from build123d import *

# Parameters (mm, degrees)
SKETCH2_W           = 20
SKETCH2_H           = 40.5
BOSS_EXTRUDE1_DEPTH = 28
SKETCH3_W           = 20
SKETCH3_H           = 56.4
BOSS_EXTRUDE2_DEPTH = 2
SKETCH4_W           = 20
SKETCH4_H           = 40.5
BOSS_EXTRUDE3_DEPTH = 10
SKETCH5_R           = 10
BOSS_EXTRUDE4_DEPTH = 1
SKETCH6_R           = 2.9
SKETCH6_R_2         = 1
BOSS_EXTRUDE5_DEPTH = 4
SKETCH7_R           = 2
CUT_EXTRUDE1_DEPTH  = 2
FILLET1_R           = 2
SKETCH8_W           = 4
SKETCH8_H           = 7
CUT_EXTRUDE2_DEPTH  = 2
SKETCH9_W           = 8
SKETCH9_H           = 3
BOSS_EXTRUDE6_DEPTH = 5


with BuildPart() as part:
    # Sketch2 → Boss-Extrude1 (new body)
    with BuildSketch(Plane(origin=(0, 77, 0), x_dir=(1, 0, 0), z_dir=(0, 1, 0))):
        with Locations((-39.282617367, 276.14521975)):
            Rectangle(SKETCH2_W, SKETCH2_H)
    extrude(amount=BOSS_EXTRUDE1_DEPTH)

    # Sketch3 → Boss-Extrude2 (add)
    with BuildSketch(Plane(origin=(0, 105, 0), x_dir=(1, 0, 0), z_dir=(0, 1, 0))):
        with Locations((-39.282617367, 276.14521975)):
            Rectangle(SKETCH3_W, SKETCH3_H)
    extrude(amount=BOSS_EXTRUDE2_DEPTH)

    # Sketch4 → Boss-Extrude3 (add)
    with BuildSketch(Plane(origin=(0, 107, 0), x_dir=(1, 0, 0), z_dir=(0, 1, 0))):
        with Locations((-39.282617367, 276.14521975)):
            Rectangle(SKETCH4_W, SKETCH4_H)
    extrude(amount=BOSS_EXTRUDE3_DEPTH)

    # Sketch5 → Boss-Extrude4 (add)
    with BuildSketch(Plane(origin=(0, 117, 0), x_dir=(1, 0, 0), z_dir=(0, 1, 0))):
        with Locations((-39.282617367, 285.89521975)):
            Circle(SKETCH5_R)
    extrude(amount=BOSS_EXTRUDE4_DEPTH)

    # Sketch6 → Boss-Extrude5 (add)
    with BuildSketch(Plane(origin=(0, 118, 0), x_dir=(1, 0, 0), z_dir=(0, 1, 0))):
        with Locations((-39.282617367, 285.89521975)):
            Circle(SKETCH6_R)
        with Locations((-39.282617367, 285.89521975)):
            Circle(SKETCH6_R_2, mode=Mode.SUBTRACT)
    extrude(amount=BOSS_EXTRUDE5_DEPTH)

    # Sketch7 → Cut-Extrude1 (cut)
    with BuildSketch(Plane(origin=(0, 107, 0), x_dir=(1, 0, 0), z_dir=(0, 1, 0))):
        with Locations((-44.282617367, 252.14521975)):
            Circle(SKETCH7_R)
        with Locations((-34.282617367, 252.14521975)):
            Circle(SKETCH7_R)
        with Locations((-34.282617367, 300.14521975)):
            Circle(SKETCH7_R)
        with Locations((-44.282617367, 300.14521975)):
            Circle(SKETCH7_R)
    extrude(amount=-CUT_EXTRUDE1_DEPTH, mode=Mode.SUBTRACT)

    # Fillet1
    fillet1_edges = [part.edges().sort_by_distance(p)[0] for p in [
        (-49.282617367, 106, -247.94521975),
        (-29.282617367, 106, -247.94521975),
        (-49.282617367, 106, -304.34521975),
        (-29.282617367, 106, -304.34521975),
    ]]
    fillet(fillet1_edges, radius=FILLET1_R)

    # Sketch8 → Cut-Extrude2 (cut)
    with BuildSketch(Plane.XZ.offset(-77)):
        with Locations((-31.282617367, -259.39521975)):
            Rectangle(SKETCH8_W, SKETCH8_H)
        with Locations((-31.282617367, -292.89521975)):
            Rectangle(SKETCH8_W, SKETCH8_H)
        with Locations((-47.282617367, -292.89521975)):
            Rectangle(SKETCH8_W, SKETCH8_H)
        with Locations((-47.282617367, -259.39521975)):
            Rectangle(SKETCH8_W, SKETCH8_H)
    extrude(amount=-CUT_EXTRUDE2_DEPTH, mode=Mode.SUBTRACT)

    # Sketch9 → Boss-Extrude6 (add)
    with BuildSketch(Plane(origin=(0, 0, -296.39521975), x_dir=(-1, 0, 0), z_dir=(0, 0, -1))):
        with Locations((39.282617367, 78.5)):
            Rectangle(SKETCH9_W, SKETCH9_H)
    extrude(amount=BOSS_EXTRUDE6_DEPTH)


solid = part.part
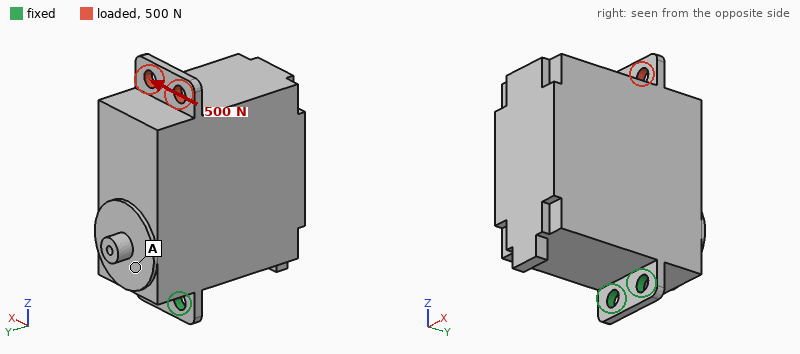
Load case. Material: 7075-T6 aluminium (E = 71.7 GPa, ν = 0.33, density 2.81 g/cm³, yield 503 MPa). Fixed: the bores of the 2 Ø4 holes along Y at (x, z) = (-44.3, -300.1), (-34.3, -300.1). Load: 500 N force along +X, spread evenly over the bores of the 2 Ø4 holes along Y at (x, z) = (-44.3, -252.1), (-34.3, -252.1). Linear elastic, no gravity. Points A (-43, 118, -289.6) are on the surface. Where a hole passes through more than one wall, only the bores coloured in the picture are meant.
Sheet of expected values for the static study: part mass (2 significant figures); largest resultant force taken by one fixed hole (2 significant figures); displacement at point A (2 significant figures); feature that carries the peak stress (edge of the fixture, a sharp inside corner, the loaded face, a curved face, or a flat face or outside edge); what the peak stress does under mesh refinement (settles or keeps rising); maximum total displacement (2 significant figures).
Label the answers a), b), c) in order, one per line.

a) 93 g
b) 1.9 kN
c) 15 µm
d) edge of the fixture
e) keeps rising
f) 96 µm
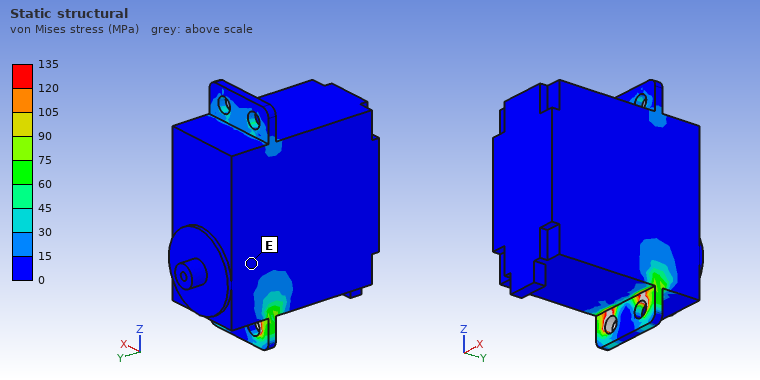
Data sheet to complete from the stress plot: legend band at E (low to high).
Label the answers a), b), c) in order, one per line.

a) 0 to 15 MPa
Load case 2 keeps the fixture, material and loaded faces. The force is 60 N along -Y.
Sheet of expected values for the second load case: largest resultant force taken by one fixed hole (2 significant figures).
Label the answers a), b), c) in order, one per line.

a) 32 N
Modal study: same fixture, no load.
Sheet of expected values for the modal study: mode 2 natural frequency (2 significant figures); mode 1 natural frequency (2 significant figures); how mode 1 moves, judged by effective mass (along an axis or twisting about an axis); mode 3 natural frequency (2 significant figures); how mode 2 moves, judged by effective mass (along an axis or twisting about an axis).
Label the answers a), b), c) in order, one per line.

a) 1900 Hz
b) 340 Hz
c) along Y
d) 3200 Hz
e) along X
